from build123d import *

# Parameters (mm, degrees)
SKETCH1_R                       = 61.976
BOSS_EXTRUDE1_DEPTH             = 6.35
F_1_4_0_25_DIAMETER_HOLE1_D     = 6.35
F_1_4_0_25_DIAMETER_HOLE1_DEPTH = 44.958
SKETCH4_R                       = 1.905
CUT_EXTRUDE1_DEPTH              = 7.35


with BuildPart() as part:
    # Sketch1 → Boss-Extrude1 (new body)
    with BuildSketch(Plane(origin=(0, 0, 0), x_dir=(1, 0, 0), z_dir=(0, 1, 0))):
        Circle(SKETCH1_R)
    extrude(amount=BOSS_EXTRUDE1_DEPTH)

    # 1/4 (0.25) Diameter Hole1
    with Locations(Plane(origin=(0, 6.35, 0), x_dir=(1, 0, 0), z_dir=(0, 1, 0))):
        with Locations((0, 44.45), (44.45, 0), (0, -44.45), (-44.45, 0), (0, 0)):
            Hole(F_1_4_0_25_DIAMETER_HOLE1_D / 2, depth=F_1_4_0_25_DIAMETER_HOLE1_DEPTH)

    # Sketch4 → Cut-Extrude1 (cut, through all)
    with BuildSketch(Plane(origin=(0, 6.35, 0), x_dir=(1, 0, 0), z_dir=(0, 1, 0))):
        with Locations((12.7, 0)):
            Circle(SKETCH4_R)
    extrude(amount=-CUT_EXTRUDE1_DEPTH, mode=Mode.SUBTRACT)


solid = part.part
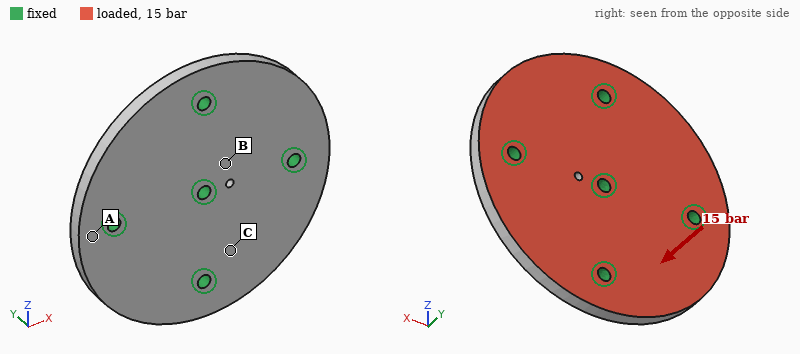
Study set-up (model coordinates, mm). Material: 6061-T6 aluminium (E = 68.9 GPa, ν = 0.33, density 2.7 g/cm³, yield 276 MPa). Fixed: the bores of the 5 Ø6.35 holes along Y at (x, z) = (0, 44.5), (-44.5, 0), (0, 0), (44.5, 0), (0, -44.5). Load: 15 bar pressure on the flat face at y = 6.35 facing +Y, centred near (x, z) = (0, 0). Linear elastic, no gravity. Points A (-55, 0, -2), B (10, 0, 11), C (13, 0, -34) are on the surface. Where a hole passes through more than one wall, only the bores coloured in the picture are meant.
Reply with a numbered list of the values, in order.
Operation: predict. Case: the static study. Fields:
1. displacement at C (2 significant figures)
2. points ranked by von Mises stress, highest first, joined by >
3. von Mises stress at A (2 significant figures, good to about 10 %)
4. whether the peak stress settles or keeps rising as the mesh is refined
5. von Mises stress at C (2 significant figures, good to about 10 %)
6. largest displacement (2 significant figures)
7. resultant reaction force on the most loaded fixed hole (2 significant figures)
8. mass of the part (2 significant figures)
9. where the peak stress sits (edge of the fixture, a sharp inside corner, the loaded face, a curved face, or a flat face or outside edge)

1. 0.029 mm
2. A > C > B
3. 66 MPa
4. keeps rising
5. 35 MPa
6. 0.14 mm
7. 3.9 kN
8. 200 g
9. edge of the fixture
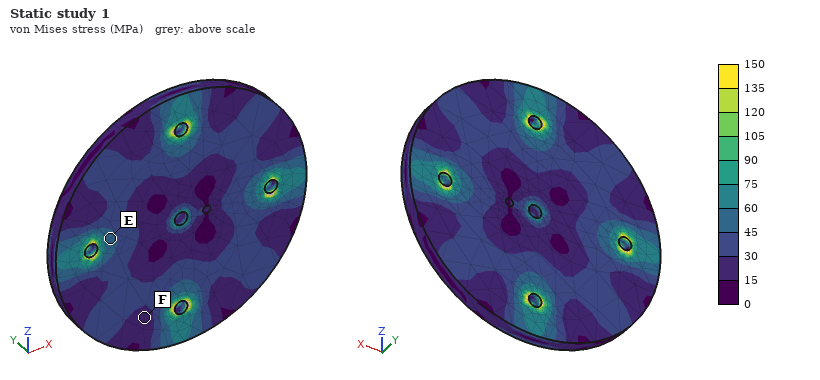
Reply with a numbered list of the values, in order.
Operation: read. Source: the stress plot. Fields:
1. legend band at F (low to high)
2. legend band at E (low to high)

1. 15 to 30 MPa
2. 45 to 60 MPa
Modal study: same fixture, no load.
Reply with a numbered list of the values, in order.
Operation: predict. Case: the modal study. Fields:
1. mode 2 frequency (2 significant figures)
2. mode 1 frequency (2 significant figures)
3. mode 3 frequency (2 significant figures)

1. 5000 Hz
2. 4600 Hz
3. 5000 Hz
